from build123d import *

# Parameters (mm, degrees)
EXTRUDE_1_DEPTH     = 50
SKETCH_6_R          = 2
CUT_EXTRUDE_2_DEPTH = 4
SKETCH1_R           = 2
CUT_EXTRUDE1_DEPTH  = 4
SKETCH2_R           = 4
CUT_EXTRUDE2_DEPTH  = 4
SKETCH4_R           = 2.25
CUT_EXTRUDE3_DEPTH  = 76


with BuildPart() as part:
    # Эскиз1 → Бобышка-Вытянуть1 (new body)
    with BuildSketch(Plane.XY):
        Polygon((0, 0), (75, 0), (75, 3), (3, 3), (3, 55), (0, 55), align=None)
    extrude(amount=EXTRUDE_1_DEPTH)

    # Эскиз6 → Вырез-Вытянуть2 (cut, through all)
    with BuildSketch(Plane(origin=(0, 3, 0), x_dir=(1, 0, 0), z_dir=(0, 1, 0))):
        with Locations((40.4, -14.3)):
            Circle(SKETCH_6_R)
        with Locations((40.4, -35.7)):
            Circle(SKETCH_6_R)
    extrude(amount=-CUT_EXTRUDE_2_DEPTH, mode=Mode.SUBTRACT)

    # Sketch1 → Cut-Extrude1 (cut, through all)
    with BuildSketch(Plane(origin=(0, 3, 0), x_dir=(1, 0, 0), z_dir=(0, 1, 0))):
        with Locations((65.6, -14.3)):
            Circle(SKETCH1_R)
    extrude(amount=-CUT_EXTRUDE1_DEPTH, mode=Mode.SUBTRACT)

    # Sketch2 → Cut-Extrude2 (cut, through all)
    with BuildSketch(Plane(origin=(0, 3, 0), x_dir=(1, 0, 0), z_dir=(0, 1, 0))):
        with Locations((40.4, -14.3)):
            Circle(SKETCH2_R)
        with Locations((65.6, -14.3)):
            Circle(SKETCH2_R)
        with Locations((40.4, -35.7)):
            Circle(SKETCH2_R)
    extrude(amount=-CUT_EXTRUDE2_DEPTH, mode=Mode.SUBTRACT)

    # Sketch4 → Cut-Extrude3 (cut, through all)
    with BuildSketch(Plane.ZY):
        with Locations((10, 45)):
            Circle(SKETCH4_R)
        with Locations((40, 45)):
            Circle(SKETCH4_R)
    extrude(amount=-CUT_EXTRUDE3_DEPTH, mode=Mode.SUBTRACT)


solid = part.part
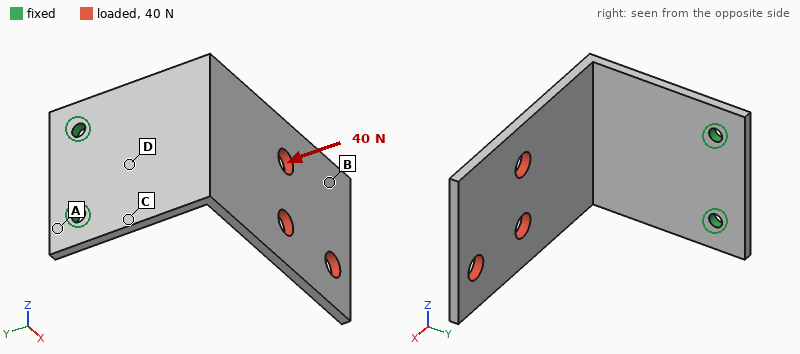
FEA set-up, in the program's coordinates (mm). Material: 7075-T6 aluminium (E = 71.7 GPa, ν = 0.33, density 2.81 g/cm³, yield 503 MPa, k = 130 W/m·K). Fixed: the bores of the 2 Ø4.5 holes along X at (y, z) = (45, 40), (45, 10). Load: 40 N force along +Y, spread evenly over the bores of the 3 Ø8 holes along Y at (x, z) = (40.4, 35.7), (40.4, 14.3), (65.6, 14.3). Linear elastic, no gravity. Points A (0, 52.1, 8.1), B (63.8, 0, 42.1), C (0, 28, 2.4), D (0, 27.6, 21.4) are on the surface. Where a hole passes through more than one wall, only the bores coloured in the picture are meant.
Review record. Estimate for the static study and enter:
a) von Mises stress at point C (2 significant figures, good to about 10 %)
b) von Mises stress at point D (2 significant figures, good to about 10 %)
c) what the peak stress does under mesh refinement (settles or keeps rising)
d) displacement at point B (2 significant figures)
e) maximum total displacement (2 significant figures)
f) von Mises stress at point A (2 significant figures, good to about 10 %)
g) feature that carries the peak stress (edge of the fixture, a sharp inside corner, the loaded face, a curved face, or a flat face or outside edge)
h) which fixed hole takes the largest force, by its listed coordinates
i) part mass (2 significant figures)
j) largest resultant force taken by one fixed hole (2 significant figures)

26 MPa
22 MPa
keeps rising
0.86 mm
1.1 mm
6.5 MPa
edge of the fixture
(45, 10)
52 g
25 N
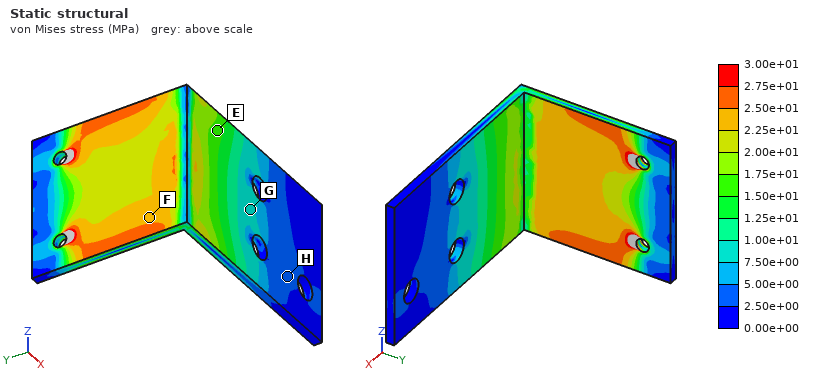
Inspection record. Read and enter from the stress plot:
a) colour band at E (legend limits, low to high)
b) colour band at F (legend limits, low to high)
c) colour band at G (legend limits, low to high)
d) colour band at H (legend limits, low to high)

1.50e+01 to 1.75e+01 MPa
2.25e+01 to 2.50e+01 MPa
7.50e+00 to 1.00e+01 MPa
2.50e+00 to 5.00e+00 MPa
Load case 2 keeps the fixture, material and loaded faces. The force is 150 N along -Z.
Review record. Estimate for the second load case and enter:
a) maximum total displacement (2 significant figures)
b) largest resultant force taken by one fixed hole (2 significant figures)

1.2 mm
290 N
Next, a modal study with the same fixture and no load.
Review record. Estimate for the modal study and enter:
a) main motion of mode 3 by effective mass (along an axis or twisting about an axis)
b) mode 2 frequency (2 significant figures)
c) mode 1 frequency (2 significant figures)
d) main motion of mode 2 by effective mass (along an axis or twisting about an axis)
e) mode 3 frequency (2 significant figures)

along X
440 Hz
240 Hz
along Z
740 Hz
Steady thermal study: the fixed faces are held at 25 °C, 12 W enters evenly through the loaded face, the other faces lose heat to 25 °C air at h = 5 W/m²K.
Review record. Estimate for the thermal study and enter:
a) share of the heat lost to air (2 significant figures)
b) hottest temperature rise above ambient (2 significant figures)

16 %
54 K
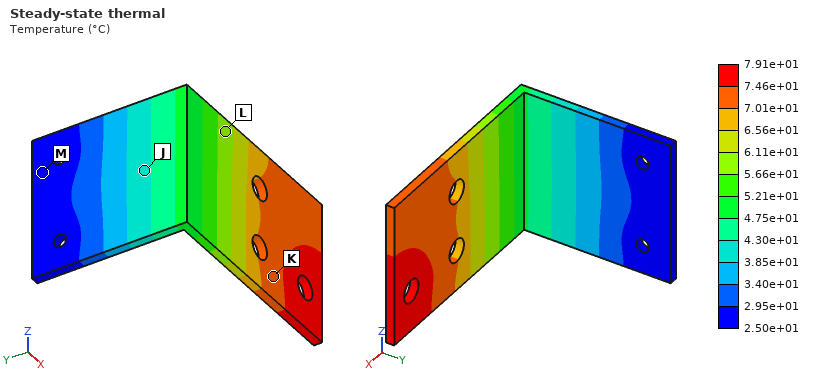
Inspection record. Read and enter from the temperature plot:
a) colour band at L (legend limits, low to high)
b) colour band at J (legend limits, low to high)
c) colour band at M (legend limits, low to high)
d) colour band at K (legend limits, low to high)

5.66e+01 to 6.11e+01 °C
3.85e+01 to 4.30e+01 °C
2.50e+01 to 2.95e+01 °C
7.01e+01 to 7.46e+01 °C
